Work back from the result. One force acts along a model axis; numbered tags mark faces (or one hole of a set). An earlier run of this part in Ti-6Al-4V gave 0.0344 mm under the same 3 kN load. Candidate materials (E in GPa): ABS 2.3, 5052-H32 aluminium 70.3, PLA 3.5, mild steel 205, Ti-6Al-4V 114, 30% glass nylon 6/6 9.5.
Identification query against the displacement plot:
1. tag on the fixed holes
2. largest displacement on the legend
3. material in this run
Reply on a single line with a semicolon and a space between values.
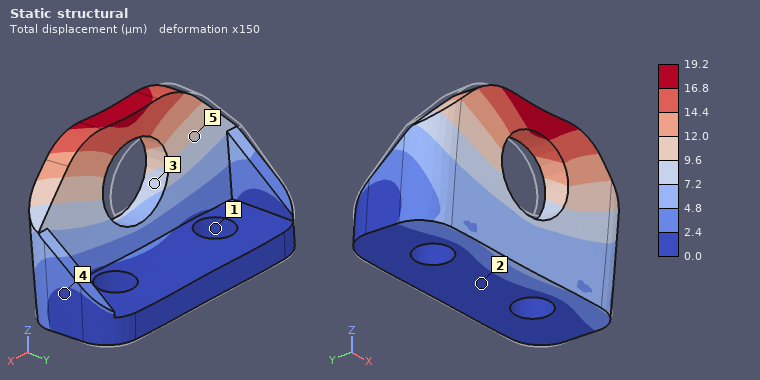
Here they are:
1; 19.2 µm; mild steel
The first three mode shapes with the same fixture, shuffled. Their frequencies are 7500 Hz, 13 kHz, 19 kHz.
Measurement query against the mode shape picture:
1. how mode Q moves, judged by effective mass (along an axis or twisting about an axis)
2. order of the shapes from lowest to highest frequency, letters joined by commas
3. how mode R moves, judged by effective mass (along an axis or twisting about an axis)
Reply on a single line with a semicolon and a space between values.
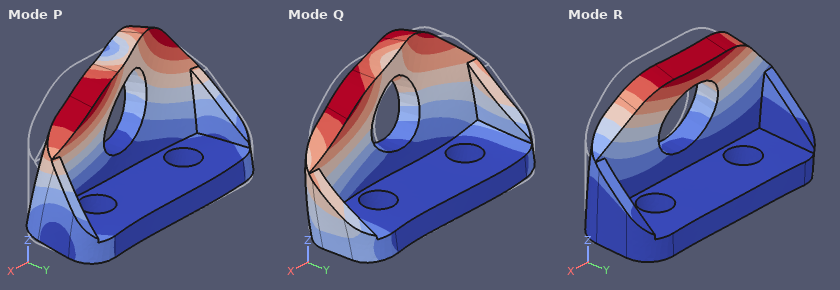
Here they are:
along X; R, P, Q; along Y
